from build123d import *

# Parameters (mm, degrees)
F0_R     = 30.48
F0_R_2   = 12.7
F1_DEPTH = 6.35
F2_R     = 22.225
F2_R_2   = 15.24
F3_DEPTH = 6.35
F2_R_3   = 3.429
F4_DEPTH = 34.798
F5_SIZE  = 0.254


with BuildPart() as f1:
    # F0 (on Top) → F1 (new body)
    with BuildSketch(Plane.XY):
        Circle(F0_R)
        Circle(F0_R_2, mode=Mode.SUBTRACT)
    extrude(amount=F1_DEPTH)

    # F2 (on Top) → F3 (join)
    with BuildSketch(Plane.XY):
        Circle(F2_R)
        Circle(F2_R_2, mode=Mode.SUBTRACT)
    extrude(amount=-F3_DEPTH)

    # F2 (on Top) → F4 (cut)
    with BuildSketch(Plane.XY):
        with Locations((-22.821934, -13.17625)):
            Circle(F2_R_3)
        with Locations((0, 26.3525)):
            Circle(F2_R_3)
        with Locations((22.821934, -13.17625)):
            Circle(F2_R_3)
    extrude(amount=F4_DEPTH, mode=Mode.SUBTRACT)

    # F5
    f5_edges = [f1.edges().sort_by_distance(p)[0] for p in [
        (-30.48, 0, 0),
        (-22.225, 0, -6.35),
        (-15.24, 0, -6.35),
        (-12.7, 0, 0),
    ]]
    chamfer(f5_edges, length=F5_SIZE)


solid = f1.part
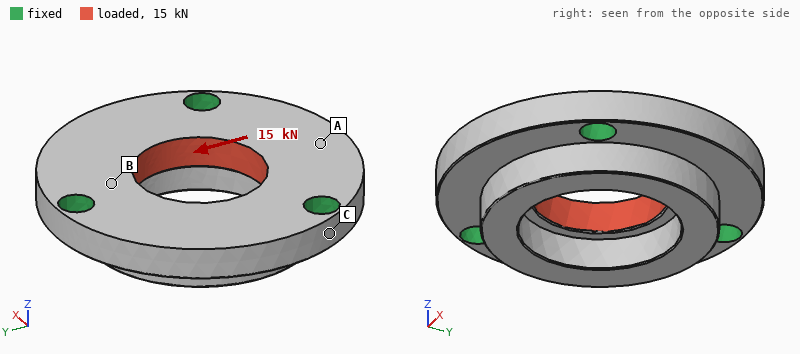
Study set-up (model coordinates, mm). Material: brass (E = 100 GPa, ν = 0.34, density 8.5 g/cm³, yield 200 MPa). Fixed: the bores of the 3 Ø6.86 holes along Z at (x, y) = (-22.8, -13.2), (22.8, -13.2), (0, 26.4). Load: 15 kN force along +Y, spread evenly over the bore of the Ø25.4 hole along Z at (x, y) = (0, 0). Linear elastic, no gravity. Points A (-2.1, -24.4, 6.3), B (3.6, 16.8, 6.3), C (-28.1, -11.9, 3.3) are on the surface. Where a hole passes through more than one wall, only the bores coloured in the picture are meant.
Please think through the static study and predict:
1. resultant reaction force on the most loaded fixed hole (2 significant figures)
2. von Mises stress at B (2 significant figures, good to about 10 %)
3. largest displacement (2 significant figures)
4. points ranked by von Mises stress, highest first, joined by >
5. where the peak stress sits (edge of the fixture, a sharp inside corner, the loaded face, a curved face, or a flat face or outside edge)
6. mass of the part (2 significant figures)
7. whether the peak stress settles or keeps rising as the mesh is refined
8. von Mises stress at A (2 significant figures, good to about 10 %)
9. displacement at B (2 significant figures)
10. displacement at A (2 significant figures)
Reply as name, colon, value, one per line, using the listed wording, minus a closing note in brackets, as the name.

resultant reaction force on the most loaded fixed hole: 5.4 kN
von Mises stress at B: 52 MPa
largest displacement: 16 µm
points ranked by von Mises stress, highest first, joined by >: B > A > C
where the peak stress sits: edge of the fixture
mass of the part: 170 g
whether the peak stress settles or keeps rising as the mesh is refined: keeps rising
von Mises stress at A: 29 MPa
displacement at B: 4.0 µm
displacement at A: 13 µm
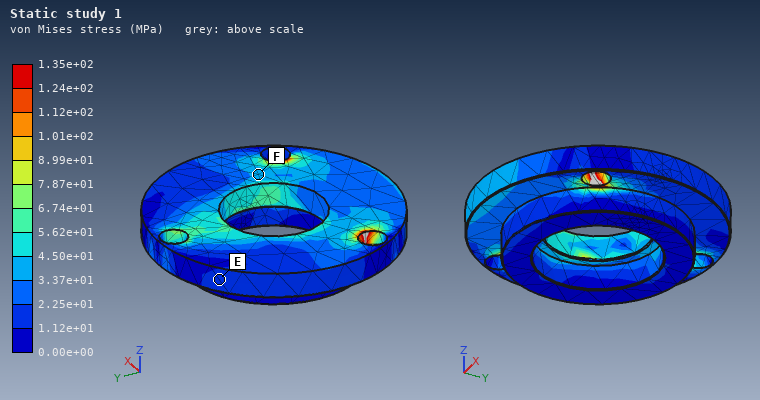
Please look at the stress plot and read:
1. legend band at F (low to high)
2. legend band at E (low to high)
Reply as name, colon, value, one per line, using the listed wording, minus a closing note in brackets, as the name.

legend band at F: 3.37e+01 to 4.50e+01 MPa
legend band at E: 1.12e+01 to 2.25e+01 MPa
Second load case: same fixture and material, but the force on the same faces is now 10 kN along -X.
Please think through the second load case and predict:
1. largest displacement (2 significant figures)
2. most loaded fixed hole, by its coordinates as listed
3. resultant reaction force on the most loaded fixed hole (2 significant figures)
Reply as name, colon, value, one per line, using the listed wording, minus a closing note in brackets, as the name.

largest displacement: 9.7 µm
most loaded fixed hole, by its coordinates as listed: (0, 26.4)
resultant reaction force on the most loaded fixed hole: 3.8 kN
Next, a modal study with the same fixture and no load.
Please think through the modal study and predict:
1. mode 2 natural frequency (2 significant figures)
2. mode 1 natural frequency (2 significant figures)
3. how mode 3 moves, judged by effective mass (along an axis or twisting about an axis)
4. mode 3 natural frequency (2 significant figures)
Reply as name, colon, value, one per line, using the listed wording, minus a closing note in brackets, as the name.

mode 2 natural frequency: 8900 Hz
mode 1 natural frequency: 8900 Hz
how mode 3 moves, judged by effective mass: along Z
mode 3 natural frequency: 11 kHz
